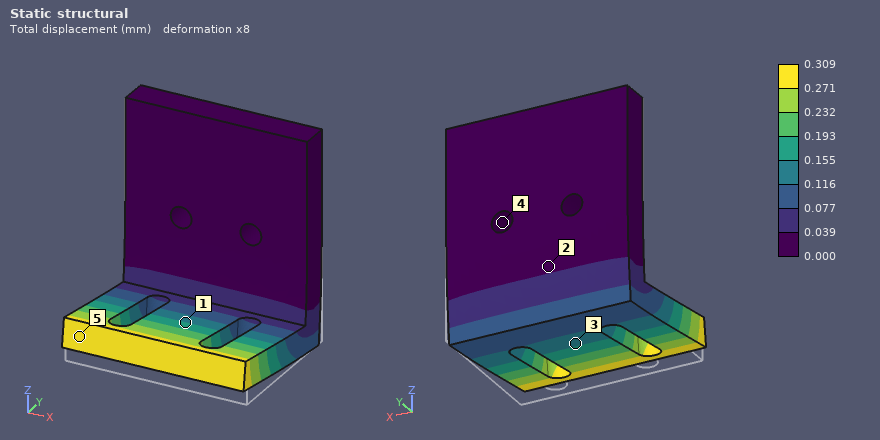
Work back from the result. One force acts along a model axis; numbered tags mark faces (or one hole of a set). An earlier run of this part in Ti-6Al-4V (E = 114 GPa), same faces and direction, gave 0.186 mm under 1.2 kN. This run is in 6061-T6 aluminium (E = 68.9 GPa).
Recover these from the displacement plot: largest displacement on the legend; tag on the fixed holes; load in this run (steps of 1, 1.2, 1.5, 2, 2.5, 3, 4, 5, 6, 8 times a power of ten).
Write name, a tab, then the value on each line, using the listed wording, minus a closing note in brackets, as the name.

largest displacement on the legend	0.309 mm
tag on the fixed holes	4
load in this run	1.2 kN
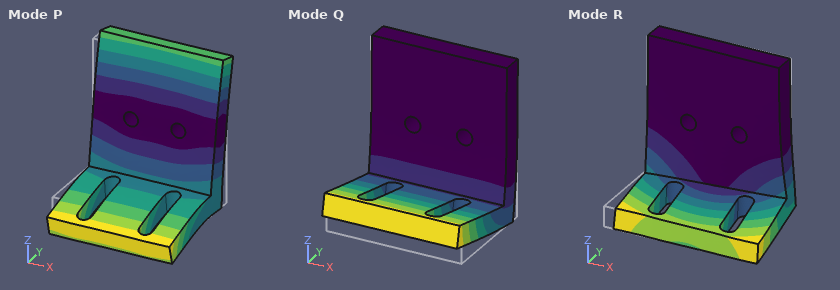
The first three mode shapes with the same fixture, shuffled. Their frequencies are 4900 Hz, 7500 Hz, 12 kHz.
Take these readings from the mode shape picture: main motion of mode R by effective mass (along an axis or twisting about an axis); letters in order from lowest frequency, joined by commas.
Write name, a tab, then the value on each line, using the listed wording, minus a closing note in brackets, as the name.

main motion of mode R by effective mass	along X
letters in order from lowest frequency, joined by commas	Q, R, P
